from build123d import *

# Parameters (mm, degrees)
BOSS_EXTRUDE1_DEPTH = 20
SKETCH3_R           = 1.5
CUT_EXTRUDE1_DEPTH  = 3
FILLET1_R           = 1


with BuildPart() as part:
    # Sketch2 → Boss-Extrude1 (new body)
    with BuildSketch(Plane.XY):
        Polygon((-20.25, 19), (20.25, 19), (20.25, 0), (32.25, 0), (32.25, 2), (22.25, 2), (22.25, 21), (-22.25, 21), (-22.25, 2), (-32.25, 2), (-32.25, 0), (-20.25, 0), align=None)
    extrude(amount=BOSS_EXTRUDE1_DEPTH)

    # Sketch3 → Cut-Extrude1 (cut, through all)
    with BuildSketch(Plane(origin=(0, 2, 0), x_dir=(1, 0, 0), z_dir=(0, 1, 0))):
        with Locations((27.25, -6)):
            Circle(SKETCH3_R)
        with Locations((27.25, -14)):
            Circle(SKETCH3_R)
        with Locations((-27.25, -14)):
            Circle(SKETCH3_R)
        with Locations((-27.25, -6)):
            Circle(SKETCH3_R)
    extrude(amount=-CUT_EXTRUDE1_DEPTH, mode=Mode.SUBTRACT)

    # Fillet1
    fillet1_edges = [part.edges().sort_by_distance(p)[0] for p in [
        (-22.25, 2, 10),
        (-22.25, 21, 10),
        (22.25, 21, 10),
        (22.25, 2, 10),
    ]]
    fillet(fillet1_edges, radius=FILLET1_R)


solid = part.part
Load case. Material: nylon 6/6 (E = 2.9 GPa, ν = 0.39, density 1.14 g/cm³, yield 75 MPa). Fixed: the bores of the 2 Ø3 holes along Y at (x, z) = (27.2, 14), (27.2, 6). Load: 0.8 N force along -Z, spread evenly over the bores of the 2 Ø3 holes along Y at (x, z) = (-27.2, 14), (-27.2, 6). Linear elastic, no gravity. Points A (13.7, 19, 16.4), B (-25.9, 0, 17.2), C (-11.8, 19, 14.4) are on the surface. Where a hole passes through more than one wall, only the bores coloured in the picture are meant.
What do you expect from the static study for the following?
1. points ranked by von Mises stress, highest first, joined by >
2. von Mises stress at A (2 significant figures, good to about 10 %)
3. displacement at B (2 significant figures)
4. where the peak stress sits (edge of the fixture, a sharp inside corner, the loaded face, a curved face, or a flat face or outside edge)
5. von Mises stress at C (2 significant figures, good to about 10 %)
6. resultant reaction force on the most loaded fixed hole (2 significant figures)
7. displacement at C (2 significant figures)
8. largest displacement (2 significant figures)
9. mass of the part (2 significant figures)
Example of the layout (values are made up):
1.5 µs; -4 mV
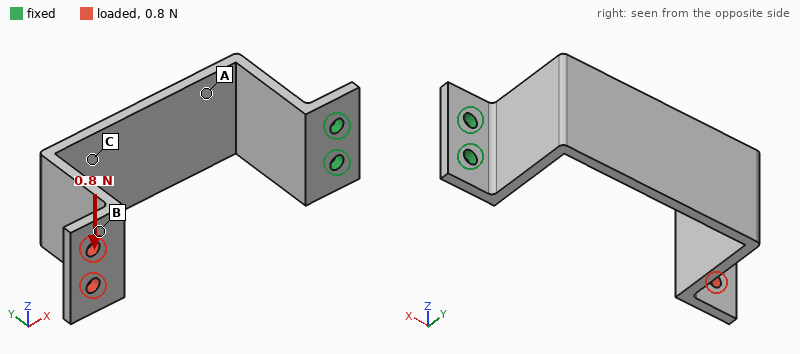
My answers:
A > C > B; 1.3 MPa; 0.76 mm; a curved face; 0.96 MPa; 4.1 N; 0.35 mm; 0.84 mm; 4.6 g
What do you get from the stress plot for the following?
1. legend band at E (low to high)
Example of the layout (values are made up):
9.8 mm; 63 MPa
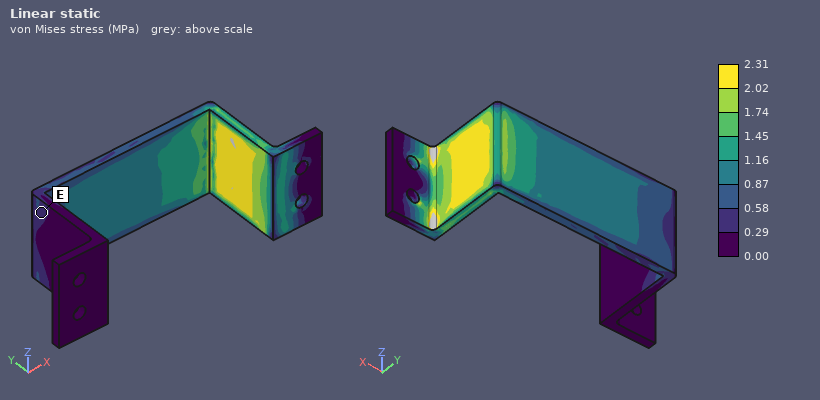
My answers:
0.29 to 0.58 MPa
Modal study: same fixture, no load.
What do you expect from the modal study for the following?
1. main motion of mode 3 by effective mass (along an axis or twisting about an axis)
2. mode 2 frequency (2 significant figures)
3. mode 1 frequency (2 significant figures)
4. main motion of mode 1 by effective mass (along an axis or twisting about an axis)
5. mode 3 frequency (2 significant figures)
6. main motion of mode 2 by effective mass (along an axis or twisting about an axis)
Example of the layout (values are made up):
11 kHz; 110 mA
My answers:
along X; 150 Hz; 84 Hz; along Y; 290 Hz; along Z
